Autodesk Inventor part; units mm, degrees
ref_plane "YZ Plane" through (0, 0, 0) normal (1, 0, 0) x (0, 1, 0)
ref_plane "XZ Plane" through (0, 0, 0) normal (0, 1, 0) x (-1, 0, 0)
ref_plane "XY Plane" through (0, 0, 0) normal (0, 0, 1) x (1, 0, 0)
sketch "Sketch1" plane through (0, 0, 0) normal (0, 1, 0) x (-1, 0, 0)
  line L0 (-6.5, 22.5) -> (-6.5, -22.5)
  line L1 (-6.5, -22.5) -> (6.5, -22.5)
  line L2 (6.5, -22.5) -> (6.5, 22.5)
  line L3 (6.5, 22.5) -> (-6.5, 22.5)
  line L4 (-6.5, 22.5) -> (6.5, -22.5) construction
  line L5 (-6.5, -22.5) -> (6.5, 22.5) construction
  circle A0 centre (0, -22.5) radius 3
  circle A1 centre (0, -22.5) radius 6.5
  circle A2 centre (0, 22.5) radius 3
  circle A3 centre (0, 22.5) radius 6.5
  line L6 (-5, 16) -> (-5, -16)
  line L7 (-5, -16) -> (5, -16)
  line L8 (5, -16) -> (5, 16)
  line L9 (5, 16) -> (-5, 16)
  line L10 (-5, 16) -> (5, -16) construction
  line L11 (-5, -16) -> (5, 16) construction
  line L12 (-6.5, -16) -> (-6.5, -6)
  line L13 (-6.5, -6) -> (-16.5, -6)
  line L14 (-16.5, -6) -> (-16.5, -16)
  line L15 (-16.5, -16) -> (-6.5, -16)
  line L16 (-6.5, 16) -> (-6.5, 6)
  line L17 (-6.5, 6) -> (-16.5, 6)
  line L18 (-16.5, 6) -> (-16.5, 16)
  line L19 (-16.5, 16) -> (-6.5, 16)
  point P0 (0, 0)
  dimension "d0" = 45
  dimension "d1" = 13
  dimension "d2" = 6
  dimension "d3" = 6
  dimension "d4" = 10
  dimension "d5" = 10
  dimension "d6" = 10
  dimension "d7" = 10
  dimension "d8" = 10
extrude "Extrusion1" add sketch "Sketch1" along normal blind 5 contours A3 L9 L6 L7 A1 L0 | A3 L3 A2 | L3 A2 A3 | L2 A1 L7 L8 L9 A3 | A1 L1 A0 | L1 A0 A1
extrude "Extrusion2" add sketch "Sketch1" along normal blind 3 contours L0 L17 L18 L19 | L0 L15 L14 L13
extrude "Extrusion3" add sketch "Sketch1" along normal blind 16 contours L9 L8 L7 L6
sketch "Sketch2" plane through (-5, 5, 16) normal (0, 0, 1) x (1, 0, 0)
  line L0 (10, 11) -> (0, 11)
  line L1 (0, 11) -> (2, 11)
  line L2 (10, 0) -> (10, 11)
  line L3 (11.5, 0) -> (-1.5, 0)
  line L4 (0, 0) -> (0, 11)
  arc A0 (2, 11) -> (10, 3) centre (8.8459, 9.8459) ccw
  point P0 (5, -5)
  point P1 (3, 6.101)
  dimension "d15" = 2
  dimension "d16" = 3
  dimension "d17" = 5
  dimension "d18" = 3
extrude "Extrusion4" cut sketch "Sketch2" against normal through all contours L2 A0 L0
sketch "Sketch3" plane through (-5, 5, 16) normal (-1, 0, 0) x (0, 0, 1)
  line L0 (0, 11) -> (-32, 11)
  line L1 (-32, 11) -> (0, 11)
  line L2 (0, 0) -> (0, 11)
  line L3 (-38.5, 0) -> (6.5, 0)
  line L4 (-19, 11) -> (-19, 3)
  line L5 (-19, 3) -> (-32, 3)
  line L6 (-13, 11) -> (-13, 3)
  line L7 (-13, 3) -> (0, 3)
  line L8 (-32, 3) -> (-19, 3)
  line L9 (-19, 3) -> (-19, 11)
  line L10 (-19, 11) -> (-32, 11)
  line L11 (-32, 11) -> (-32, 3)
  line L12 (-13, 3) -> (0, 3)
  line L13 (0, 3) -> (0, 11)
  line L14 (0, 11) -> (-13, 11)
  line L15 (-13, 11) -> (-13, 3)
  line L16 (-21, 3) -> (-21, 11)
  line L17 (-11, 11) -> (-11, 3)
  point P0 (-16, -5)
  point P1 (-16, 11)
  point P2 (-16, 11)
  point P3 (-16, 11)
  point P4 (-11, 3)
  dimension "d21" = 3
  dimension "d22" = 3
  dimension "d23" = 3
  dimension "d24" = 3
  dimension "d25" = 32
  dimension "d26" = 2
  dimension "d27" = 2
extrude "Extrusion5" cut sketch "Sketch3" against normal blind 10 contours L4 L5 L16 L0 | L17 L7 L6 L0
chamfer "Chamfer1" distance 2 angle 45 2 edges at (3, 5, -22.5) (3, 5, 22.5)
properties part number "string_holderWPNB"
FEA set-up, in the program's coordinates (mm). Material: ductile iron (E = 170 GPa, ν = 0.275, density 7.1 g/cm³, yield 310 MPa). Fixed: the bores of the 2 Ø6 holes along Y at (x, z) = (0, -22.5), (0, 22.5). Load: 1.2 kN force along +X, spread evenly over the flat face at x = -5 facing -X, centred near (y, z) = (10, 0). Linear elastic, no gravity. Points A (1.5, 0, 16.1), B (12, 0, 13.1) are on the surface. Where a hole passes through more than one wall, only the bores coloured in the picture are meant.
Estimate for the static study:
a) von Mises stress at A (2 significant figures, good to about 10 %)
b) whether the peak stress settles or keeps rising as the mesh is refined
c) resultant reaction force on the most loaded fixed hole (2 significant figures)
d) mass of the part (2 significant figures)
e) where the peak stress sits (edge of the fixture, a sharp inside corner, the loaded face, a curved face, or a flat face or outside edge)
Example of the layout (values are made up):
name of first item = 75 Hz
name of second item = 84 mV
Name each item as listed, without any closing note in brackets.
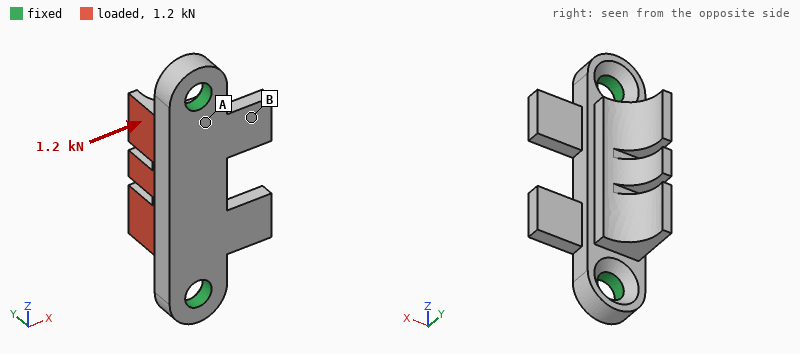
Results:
von Mises stress at A = 39 MPa
whether the peak stress settles or keeps rising as the mesh is refined = keeps rising
resultant reaction force on the most loaded fixed hole = 600 N
mass of the part = 39 g
where the peak stress sits = edge of the fixture
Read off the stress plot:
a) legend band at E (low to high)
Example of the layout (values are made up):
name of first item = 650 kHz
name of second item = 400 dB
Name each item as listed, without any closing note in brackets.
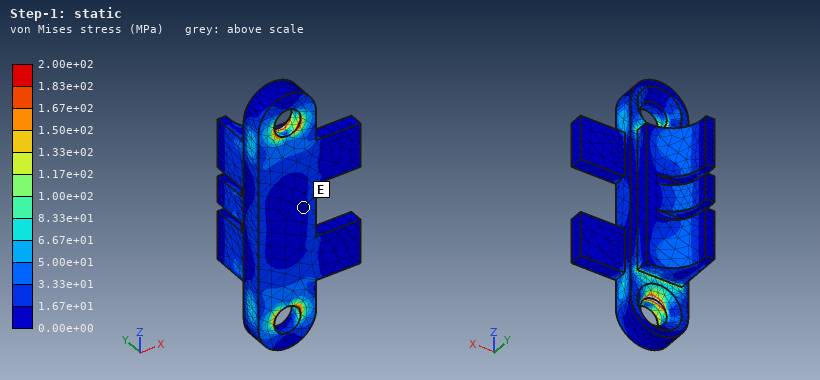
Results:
legend band at E = 0.00e+00 to 1.67e+01 MPa
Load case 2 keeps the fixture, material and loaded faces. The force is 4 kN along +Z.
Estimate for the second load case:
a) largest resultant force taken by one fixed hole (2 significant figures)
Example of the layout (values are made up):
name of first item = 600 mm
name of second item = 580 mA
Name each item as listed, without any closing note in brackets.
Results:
largest resultant force taken by one fixed hole = 2.2 kN
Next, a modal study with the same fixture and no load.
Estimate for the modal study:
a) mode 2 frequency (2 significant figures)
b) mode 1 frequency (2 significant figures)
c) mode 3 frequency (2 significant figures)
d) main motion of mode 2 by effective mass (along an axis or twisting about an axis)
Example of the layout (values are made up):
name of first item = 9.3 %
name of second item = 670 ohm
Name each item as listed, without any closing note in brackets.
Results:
mode 2 frequency = 12 kHz
mode 1 frequency = 9600 Hz
mode 3 frequency = 15 kHz
main motion of mode 2 by effective mass = along Y
